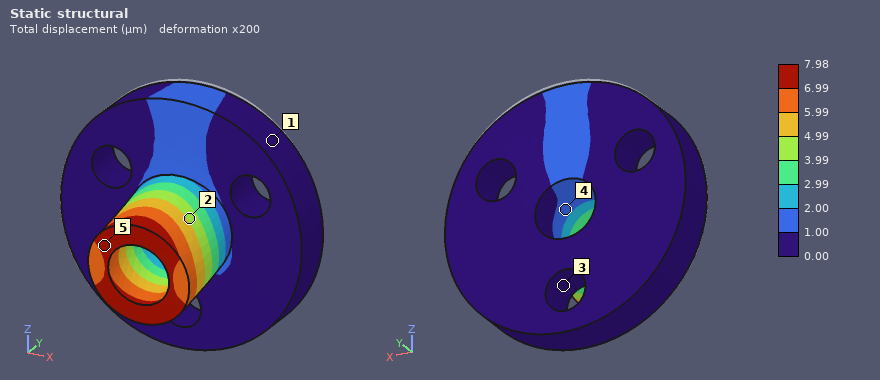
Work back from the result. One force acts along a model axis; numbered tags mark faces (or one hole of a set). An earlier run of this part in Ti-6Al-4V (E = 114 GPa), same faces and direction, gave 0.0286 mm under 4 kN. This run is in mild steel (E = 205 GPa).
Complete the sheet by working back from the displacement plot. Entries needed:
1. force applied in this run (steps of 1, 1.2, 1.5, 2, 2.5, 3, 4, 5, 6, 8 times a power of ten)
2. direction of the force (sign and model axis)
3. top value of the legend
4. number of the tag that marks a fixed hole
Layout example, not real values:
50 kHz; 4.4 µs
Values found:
2 kN; -Z; 7.98 µm; 3
